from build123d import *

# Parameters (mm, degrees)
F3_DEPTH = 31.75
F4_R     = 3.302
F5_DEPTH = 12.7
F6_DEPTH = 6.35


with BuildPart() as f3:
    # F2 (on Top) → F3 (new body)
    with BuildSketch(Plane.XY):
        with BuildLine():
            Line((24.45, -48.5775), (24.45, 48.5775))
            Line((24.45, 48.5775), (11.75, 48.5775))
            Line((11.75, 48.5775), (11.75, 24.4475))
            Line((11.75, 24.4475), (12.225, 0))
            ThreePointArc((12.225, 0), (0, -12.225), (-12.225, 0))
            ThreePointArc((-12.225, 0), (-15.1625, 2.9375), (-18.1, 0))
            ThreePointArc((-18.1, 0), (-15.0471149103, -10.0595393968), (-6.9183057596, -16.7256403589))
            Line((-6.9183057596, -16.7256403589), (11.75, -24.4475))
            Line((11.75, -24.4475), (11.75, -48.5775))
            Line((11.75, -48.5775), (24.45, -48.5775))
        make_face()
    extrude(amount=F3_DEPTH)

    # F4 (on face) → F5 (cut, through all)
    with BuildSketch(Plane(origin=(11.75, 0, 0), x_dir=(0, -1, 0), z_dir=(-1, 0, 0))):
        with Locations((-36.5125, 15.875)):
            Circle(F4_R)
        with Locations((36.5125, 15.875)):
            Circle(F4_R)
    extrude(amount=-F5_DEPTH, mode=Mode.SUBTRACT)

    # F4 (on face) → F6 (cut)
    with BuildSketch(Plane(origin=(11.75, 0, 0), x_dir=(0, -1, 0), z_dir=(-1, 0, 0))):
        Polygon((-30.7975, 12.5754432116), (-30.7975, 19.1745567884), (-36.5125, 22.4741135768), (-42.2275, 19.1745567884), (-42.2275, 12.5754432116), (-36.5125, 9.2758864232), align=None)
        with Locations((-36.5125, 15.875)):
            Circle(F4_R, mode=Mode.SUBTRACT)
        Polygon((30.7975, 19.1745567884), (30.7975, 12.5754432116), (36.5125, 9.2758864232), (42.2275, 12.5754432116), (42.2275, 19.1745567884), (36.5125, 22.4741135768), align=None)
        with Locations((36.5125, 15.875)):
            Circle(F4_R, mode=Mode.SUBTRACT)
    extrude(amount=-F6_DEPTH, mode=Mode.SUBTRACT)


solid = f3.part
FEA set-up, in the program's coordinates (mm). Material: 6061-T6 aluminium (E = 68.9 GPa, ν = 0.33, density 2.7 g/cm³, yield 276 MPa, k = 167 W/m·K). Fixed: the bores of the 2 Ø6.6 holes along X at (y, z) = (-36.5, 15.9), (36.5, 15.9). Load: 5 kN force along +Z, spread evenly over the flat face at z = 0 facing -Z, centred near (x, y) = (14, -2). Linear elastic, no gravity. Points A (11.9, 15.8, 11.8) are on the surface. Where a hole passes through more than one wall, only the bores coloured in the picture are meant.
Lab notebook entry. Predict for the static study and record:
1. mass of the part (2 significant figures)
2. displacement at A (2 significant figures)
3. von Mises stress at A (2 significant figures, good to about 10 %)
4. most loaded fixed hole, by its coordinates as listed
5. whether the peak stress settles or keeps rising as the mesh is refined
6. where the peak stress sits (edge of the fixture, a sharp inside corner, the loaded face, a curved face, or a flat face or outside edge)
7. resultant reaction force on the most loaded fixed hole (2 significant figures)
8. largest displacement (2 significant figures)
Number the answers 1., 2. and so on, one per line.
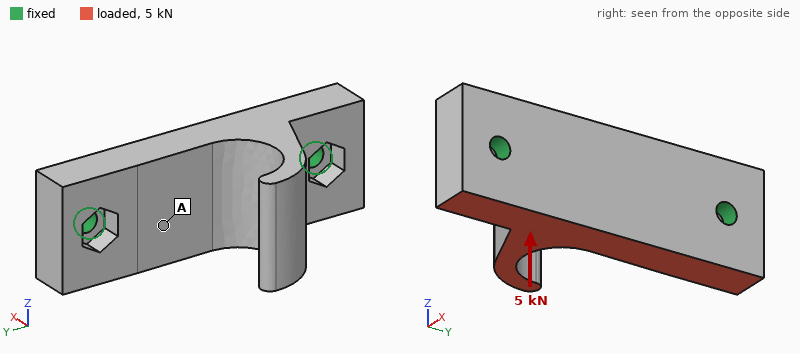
1. 130 g
2. 20 µm
3. 16 MPa
4. (-36.5, 15.9)
5. keeps rising
6. edge of the fixture
7. 2.7 kN
8. 87 µm
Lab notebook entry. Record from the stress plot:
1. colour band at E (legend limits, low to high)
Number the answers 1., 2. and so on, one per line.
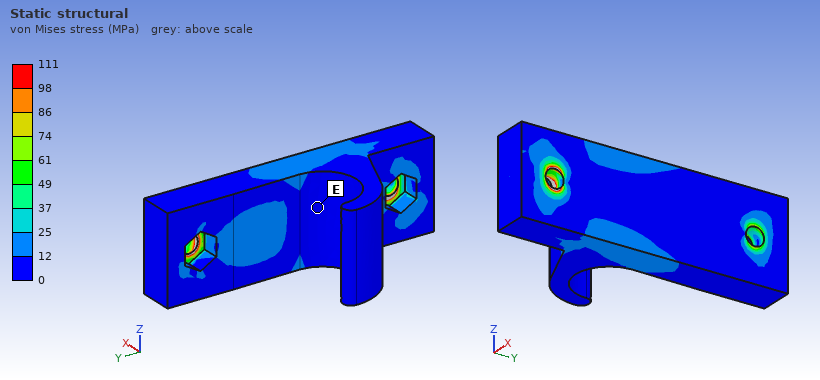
1. 0 to 12 MPa
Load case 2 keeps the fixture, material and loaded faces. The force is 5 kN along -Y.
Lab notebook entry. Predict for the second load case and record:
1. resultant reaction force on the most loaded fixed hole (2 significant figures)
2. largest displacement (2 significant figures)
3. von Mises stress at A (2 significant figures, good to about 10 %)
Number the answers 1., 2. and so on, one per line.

1. 2.9 kN
2. 70 µm
3. 5.8 MPa
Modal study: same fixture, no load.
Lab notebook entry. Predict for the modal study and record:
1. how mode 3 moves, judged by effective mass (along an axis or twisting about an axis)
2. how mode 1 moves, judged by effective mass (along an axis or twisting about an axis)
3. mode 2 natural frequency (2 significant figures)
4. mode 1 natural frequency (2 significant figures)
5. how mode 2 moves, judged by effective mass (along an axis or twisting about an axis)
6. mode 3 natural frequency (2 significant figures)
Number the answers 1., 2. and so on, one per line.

1. along X
2. along Z
3. 4900 Hz
4. 4200 Hz
5. along X
6. 8300 Hz
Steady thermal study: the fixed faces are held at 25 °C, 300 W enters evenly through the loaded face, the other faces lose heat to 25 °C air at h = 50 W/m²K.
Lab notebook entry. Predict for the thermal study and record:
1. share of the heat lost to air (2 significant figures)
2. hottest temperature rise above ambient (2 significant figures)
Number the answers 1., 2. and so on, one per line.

1. 6.6 %
2. 76 K
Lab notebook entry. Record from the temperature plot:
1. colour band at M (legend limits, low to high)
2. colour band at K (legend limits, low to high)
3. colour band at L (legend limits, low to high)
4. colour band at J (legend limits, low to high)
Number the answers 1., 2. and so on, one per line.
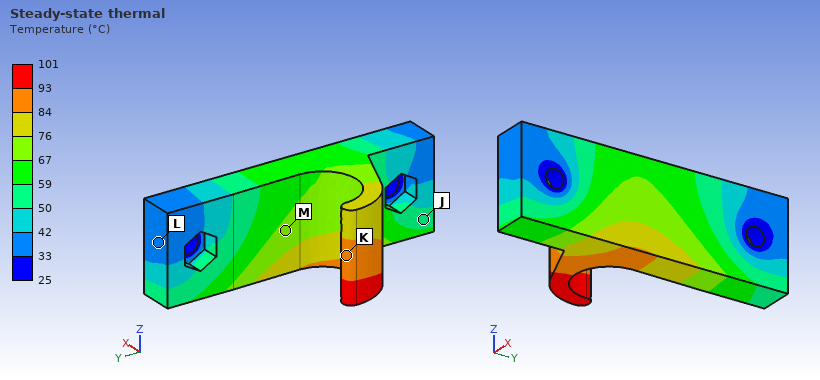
1. 67 to 76 °C
2. 84 to 93 °C
3. 33 to 42 °C
4. 50 to 59 °C
